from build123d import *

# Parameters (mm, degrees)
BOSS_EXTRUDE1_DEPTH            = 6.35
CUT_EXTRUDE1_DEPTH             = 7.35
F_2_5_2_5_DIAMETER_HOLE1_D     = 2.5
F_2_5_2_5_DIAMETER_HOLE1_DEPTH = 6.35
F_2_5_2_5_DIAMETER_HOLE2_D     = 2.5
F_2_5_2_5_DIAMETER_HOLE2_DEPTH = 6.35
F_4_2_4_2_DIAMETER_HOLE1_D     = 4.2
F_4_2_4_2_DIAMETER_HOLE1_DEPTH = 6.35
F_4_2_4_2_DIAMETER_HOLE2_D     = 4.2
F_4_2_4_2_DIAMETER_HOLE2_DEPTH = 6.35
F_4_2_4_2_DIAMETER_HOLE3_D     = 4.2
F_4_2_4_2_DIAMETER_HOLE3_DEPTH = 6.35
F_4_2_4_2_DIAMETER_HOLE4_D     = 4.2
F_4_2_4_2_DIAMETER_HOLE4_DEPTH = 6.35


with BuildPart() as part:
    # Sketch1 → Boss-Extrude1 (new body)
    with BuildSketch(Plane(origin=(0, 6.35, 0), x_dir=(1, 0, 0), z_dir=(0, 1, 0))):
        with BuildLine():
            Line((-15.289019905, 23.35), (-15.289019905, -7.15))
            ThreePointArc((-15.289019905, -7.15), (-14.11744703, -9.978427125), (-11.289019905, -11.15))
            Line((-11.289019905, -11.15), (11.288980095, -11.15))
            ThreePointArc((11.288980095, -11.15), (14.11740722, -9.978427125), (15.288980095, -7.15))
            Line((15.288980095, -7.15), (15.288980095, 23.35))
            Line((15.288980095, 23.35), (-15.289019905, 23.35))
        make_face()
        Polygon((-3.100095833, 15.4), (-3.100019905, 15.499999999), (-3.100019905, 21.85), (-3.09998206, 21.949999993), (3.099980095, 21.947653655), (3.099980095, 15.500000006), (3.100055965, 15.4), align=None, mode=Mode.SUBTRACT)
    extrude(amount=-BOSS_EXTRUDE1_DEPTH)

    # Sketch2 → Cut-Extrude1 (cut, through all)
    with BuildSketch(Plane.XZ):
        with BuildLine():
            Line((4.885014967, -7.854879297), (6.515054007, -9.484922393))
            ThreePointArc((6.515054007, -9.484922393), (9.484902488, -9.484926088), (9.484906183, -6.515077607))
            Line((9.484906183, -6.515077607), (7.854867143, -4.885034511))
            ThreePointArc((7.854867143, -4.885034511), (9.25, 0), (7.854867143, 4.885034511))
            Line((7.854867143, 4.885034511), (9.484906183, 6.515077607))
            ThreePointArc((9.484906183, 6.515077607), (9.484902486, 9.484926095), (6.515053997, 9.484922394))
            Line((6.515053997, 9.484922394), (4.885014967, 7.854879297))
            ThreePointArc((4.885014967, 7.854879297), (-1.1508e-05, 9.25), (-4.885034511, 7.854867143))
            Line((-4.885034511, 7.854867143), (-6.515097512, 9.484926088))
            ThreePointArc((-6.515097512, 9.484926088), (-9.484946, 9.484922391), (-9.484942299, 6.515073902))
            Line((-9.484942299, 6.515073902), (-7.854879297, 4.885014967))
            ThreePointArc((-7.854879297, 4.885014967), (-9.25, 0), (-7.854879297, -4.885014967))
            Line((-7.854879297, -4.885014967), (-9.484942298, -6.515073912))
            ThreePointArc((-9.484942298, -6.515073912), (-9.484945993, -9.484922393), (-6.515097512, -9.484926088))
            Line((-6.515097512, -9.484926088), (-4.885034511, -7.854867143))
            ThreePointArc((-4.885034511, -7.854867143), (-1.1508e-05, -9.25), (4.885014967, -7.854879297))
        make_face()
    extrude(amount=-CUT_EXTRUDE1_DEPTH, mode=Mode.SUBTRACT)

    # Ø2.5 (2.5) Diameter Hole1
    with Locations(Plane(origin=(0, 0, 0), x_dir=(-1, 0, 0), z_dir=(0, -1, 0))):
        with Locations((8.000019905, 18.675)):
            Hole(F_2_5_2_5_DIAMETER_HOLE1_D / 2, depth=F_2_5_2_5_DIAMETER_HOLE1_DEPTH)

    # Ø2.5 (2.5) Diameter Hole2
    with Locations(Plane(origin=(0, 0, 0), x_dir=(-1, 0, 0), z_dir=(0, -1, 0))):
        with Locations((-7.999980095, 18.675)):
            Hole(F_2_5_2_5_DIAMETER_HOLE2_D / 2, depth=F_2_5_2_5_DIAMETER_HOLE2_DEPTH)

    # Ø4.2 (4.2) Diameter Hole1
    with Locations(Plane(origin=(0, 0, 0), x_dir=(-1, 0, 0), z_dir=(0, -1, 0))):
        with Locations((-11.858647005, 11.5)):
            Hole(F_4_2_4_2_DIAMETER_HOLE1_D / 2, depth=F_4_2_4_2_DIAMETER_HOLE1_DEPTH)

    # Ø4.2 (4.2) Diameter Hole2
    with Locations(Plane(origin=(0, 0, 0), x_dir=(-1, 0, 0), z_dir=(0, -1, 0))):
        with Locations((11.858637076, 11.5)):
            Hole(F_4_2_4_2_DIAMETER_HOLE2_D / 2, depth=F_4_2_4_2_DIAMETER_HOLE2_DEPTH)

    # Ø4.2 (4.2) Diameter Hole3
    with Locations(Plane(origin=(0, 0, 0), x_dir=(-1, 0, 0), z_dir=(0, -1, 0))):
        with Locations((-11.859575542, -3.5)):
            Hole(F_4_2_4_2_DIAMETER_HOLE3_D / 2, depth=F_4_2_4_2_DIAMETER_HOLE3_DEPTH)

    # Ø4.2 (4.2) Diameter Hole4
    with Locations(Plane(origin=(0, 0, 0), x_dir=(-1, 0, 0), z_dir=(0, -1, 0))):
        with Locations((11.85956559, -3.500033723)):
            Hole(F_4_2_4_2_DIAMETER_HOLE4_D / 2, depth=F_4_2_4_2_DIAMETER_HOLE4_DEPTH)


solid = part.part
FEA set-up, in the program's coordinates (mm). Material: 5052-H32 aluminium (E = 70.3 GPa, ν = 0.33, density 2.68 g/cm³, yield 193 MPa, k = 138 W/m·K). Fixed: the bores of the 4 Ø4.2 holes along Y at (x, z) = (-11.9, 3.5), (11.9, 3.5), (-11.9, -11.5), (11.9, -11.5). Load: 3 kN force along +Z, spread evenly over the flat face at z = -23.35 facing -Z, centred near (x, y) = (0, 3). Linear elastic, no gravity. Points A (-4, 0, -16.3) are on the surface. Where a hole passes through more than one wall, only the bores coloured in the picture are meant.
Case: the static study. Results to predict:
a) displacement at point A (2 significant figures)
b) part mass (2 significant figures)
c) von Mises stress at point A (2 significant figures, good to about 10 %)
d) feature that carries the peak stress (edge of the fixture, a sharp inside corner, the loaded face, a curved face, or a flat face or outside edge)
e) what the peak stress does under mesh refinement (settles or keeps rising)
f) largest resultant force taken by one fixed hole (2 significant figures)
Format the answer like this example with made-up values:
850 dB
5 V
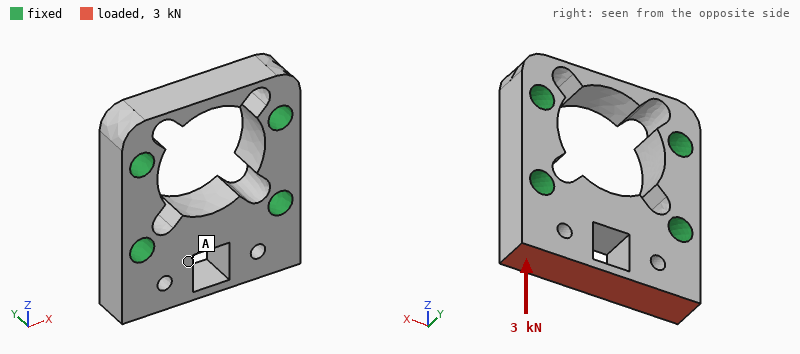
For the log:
4.9 µm
10 g
17 MPa
a sharp inside corner
keeps rising
1.5 kN
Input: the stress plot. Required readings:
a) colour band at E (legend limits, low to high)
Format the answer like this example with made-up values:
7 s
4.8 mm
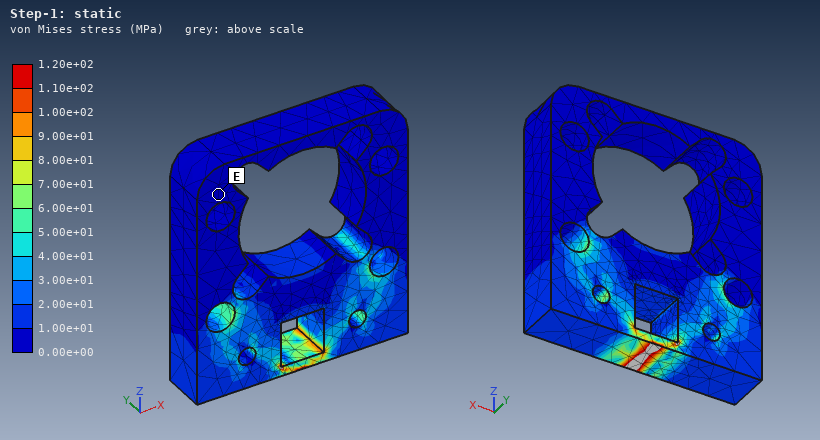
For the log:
0.00e+00 to 1.00e+01 MPa
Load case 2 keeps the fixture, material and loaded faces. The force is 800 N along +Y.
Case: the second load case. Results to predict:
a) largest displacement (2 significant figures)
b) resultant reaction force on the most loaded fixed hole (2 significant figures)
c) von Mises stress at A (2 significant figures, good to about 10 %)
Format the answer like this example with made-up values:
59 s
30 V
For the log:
23 µm
400 N
26 MPa
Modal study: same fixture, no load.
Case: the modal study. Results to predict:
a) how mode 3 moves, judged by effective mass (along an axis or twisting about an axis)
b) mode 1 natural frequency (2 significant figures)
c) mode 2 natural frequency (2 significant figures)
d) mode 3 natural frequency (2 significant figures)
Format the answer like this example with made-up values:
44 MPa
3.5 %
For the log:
along Y
17 kHz
27 kHz
28 kHz
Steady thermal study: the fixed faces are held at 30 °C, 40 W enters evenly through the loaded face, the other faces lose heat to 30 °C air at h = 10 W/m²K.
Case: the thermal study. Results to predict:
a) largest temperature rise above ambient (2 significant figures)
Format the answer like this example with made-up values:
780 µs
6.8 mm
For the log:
34 K
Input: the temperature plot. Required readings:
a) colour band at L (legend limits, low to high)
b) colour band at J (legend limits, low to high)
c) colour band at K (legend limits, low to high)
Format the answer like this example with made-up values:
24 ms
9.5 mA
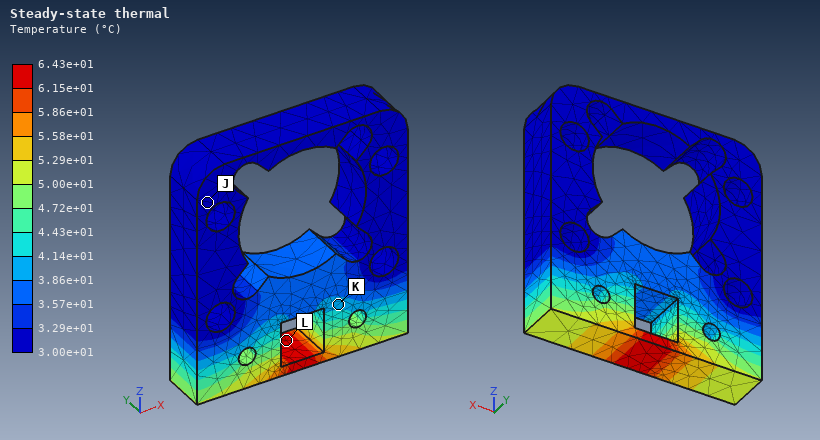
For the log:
6.15e+01 to 6.43e+01 °C
3.00e+01 to 3.29e+01 °C
3.86e+01 to 4.14e+01 °C
